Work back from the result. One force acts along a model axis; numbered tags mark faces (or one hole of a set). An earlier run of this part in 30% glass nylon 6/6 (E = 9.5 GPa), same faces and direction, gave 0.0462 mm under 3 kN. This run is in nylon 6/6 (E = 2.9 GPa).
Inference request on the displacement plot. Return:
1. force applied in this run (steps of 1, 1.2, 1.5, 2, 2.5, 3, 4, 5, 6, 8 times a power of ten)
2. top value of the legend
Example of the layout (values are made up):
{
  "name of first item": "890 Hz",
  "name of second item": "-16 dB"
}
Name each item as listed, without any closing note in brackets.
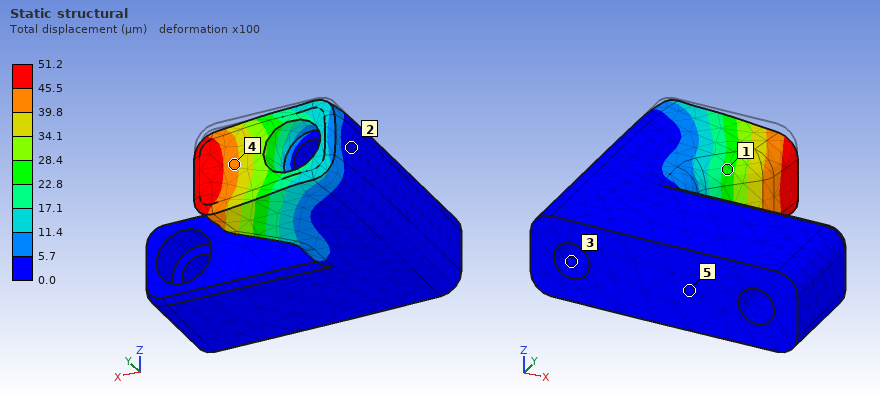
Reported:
{
  "force applied in this run": "1 kN",
  "top value of the legend": "51.2 µm"
}
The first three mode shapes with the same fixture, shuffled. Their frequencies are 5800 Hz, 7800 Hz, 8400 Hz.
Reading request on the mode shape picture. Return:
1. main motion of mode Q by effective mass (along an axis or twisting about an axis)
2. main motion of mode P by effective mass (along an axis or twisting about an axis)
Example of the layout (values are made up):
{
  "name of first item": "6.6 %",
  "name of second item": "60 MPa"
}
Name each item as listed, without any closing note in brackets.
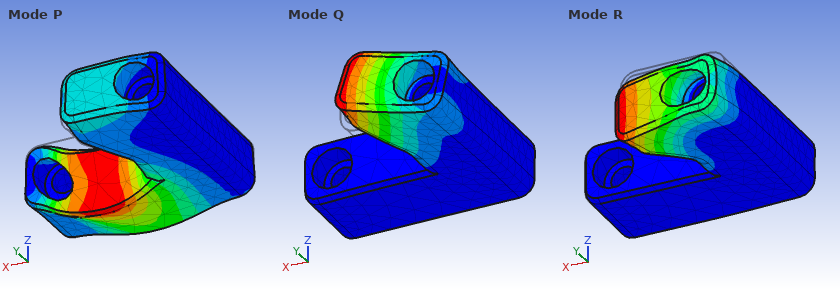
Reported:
{
  "main motion of mode Q by effective mass": "along Z",
  "main motion of mode P by effective mass": "along Z"
}
